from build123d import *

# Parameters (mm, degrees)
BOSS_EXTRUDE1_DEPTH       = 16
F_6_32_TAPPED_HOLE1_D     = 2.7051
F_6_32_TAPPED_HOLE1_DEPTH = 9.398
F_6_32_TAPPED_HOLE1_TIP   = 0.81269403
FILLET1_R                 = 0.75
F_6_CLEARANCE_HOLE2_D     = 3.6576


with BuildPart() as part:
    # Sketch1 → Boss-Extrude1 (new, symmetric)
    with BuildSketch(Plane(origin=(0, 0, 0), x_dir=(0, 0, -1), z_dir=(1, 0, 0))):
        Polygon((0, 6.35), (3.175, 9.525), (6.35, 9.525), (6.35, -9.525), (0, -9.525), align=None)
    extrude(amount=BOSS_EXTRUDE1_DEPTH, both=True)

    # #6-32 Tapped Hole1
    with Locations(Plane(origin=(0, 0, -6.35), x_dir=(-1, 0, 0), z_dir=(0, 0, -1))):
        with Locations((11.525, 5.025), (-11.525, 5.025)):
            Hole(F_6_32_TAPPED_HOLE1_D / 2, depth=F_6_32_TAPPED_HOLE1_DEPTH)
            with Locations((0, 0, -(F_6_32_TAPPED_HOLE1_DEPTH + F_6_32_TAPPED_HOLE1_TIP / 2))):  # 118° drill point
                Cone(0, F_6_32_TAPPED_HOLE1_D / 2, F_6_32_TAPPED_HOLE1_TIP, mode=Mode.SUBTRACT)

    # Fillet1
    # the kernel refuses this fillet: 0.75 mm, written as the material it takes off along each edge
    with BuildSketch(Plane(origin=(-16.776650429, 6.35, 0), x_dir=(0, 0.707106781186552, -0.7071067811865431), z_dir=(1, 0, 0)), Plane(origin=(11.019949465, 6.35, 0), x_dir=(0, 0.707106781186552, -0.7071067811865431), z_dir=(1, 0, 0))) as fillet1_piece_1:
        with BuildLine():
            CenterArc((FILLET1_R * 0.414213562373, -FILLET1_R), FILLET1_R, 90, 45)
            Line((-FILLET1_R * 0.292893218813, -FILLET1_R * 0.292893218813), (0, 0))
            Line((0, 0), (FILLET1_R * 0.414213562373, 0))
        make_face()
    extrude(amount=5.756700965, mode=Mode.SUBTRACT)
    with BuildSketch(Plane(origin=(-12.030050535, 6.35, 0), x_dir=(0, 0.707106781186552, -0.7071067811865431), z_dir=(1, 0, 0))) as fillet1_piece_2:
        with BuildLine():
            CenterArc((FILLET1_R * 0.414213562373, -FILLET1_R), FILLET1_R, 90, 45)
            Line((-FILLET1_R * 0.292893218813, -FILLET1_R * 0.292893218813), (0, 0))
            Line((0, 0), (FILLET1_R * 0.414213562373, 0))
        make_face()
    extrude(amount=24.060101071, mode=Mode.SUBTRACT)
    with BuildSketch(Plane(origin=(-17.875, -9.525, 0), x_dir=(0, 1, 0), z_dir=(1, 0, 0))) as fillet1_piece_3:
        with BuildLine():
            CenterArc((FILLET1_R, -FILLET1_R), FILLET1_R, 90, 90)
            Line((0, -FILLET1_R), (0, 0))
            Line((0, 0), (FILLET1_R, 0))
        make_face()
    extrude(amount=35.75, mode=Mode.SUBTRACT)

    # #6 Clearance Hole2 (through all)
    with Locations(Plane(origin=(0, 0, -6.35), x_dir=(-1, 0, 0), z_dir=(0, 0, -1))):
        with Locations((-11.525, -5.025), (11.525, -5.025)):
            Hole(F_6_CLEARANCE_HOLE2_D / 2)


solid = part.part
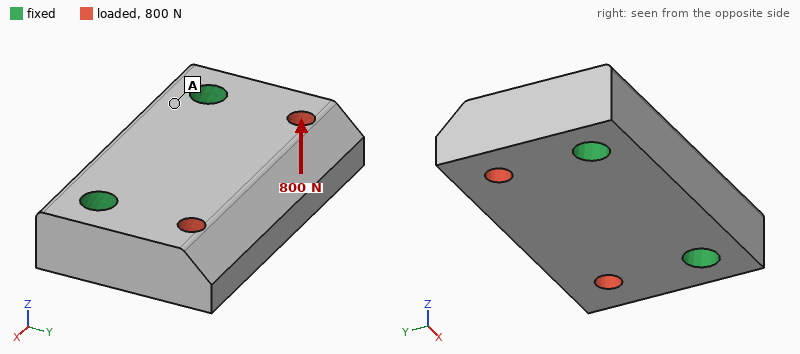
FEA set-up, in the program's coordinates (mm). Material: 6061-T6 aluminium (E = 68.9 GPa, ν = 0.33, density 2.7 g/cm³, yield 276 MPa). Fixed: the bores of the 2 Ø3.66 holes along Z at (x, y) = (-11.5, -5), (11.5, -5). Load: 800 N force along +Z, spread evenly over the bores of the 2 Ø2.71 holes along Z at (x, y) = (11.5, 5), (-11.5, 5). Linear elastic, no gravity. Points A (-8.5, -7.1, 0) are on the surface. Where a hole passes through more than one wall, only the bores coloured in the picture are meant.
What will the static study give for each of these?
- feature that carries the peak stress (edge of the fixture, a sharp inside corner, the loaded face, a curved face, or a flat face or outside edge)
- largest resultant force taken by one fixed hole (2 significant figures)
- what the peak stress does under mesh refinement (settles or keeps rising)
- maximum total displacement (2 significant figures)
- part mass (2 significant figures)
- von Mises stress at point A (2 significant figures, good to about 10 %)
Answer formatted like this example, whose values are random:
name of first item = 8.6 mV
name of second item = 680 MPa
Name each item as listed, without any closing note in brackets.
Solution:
feature that carries the peak stress = edge of the fixture
largest resultant force taken by one fixed hole = 400 N
what the peak stress does under mesh refinement = keeps rising
maximum total displacement = 15 µm
part mass = 9.4 g
von Mises stress at point A = 18 MPa
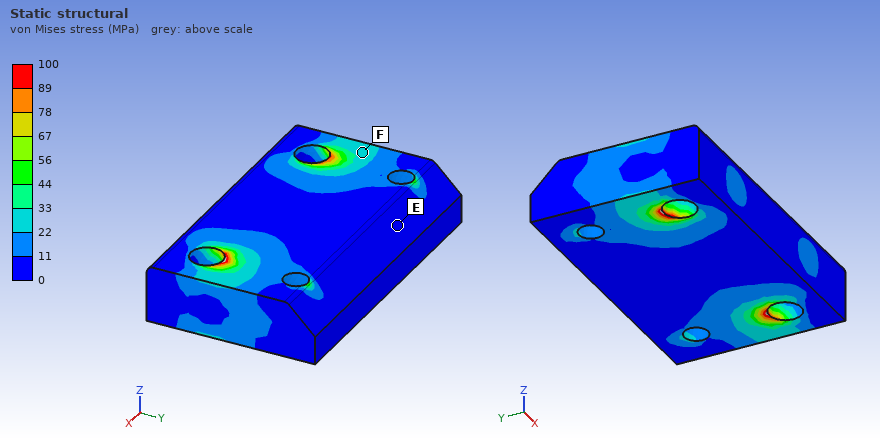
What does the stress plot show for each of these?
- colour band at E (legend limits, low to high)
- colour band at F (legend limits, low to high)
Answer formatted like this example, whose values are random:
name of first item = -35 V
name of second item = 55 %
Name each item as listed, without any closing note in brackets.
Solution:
colour band at E = 0 to 11 MPa
colour band at F = 22 to 33 MPa
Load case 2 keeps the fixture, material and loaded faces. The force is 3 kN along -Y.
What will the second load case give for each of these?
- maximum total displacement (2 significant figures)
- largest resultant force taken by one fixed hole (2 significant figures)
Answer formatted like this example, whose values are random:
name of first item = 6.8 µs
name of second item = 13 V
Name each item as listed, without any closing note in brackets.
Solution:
maximum total displacement = 8.5 µm
largest resultant force taken by one fixed hole = 1.5 kN
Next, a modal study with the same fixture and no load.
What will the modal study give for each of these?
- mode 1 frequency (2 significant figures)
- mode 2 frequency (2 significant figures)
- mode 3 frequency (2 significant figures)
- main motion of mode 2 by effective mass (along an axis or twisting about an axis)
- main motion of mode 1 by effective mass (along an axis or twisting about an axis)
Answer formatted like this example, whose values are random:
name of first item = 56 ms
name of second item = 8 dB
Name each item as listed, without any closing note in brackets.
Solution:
mode 1 frequency = 20 kHz
mode 2 frequency = 33 kHz
mode 3 frequency = 44 kHz
main motion of mode 2 by effective mass = twisting about Y
main motion of mode 1 by effective mass = along Z
